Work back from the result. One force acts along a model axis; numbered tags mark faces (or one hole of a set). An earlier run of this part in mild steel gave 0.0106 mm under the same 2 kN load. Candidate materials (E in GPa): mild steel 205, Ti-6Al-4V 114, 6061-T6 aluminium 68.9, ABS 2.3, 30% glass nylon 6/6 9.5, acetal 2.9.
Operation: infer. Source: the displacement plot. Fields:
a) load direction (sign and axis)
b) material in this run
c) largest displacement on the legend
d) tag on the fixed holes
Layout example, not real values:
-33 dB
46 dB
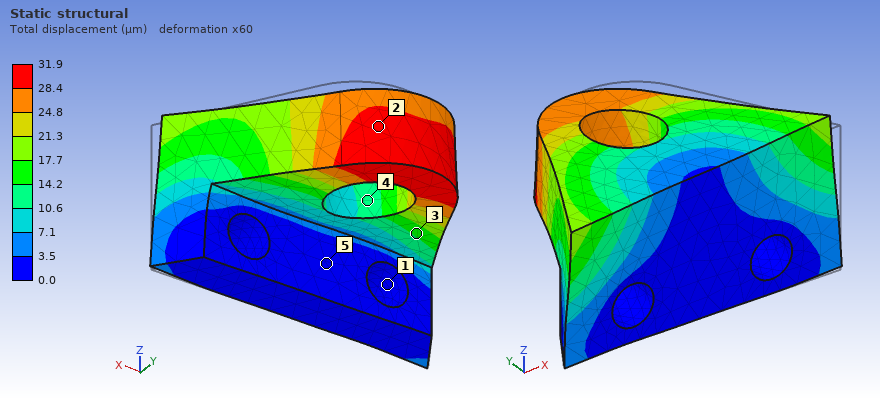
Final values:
-X
6061-T6 aluminium
31.9 µm
1
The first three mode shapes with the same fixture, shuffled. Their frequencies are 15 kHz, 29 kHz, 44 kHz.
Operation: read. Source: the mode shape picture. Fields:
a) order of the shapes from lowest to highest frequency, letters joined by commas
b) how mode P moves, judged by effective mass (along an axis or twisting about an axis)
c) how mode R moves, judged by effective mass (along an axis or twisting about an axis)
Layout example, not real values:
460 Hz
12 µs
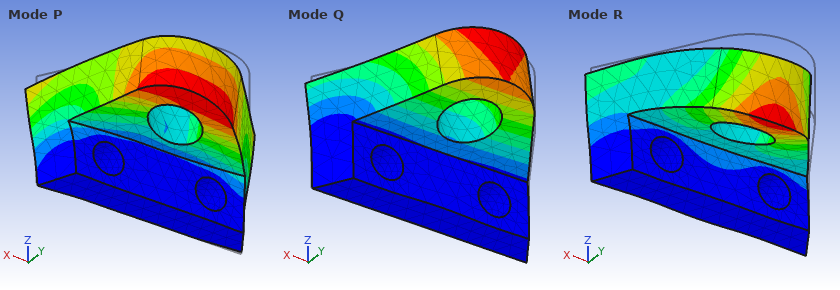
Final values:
Q, P, R
along X
along Y
